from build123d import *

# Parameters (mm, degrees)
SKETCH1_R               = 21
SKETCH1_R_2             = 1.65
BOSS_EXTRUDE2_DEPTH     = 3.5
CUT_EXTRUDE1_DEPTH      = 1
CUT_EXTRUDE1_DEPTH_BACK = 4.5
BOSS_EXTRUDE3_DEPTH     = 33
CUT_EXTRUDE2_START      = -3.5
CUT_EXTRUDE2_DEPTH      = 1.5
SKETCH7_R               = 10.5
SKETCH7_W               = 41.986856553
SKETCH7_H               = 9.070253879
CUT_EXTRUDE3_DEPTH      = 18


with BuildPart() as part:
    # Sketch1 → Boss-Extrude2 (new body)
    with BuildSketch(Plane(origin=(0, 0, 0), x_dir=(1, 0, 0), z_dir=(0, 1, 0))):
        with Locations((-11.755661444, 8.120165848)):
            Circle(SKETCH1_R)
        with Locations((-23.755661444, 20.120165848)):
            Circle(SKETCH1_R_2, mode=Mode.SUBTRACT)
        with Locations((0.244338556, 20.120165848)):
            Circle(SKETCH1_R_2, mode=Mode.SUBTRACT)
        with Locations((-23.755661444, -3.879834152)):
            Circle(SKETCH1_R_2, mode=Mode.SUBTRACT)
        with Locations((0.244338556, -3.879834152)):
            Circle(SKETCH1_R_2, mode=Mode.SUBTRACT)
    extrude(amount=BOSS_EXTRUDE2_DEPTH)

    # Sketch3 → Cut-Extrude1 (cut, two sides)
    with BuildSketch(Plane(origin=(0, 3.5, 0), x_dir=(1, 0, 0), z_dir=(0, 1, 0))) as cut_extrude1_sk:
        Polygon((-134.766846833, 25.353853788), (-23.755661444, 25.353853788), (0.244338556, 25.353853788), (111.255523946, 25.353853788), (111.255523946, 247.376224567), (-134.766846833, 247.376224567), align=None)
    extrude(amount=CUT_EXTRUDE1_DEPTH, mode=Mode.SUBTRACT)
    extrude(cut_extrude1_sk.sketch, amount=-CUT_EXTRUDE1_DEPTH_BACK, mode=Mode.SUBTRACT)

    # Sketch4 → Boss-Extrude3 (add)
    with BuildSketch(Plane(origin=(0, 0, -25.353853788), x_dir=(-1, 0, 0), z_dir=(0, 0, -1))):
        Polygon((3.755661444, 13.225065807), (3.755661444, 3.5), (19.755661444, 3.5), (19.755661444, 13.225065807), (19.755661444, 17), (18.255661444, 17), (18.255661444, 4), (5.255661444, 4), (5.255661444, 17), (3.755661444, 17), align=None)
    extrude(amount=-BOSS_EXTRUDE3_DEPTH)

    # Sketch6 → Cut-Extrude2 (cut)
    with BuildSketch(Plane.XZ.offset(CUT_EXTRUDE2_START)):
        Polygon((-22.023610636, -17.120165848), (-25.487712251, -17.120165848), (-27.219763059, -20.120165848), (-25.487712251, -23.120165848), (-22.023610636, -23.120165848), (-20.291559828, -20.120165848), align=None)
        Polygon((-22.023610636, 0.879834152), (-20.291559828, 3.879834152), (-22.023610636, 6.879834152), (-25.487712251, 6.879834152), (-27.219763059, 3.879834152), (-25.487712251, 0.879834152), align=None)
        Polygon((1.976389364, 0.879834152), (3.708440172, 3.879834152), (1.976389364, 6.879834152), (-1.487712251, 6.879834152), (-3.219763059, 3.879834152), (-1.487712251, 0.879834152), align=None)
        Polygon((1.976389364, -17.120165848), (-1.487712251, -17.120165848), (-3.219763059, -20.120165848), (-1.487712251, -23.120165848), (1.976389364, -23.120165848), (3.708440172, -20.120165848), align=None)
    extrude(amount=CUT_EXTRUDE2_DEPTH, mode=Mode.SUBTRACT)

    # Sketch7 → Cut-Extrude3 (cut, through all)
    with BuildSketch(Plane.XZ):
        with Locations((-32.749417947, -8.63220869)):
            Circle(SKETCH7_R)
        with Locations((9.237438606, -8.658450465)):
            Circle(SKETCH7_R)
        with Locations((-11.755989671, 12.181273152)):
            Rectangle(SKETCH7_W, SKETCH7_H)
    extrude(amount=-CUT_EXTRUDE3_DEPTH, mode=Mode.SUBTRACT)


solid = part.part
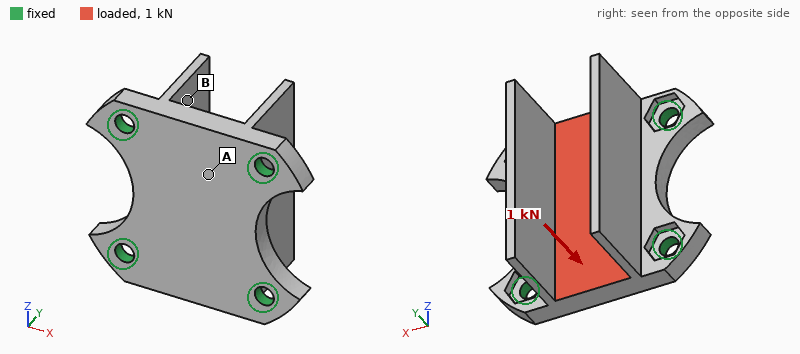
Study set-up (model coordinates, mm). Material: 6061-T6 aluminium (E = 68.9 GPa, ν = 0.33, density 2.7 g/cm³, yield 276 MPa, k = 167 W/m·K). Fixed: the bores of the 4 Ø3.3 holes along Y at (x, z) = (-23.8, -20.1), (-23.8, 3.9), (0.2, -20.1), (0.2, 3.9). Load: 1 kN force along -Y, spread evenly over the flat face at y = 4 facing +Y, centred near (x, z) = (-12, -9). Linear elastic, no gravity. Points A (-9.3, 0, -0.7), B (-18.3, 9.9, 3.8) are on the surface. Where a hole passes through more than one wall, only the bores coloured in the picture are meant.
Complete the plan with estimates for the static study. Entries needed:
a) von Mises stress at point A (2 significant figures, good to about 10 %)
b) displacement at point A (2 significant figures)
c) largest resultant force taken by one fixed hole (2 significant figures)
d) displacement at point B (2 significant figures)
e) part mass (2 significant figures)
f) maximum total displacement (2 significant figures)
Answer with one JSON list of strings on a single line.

["20 MPa", "10 µm", "350 N", "11 µm", "12 g", "18 µm"]
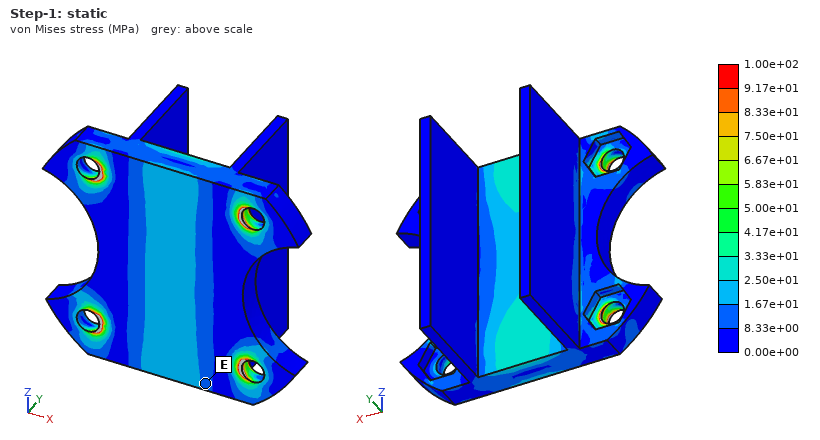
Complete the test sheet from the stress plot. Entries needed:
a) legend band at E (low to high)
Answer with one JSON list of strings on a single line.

["8.33e+00 to 1.67e+01 MPa"]
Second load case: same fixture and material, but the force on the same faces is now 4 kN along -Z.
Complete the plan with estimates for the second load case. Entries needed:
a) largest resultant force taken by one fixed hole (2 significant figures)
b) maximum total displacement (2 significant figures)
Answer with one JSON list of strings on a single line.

["1.1 kN", "20 µm"]
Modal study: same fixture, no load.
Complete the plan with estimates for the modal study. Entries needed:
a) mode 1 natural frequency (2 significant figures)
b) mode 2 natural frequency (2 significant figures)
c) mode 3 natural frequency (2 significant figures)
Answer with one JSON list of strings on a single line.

["6500 Hz", "6700 Hz", "8900 Hz"]
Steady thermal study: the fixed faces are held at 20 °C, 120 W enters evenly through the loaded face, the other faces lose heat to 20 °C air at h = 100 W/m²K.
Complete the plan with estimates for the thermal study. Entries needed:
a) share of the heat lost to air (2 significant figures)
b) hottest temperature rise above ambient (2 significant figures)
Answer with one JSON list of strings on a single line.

["7.8 %", "44 K"]
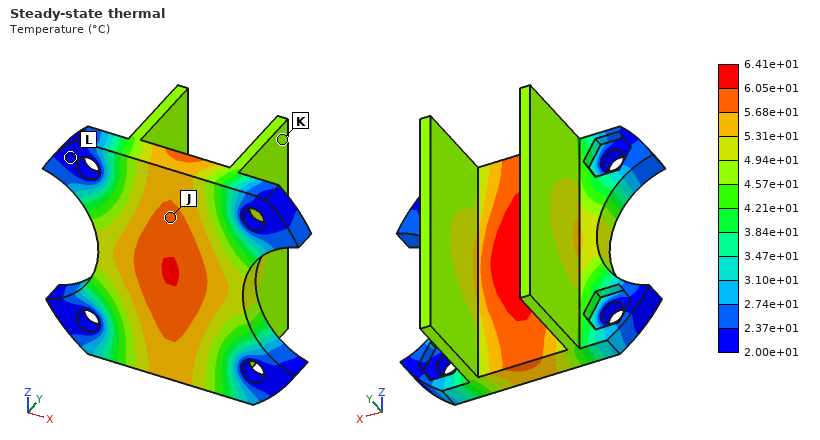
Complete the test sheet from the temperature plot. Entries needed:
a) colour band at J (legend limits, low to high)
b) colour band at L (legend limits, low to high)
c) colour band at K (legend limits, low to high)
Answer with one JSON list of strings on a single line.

["5.68e+01 to 6.05e+01 °C", "2.00e+01 to 2.37e+01 °C", "4.57e+01 to 4.94e+01 °C"]
